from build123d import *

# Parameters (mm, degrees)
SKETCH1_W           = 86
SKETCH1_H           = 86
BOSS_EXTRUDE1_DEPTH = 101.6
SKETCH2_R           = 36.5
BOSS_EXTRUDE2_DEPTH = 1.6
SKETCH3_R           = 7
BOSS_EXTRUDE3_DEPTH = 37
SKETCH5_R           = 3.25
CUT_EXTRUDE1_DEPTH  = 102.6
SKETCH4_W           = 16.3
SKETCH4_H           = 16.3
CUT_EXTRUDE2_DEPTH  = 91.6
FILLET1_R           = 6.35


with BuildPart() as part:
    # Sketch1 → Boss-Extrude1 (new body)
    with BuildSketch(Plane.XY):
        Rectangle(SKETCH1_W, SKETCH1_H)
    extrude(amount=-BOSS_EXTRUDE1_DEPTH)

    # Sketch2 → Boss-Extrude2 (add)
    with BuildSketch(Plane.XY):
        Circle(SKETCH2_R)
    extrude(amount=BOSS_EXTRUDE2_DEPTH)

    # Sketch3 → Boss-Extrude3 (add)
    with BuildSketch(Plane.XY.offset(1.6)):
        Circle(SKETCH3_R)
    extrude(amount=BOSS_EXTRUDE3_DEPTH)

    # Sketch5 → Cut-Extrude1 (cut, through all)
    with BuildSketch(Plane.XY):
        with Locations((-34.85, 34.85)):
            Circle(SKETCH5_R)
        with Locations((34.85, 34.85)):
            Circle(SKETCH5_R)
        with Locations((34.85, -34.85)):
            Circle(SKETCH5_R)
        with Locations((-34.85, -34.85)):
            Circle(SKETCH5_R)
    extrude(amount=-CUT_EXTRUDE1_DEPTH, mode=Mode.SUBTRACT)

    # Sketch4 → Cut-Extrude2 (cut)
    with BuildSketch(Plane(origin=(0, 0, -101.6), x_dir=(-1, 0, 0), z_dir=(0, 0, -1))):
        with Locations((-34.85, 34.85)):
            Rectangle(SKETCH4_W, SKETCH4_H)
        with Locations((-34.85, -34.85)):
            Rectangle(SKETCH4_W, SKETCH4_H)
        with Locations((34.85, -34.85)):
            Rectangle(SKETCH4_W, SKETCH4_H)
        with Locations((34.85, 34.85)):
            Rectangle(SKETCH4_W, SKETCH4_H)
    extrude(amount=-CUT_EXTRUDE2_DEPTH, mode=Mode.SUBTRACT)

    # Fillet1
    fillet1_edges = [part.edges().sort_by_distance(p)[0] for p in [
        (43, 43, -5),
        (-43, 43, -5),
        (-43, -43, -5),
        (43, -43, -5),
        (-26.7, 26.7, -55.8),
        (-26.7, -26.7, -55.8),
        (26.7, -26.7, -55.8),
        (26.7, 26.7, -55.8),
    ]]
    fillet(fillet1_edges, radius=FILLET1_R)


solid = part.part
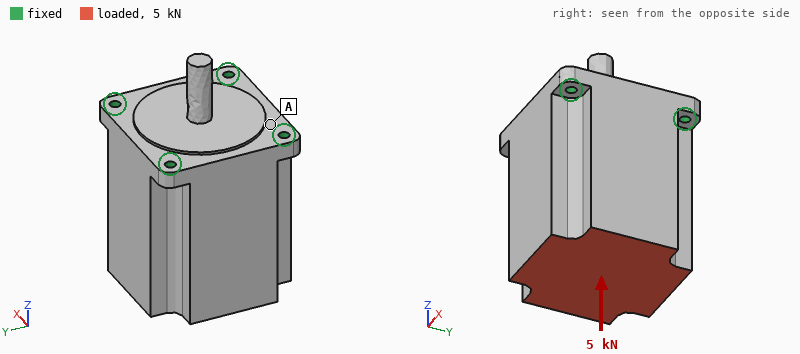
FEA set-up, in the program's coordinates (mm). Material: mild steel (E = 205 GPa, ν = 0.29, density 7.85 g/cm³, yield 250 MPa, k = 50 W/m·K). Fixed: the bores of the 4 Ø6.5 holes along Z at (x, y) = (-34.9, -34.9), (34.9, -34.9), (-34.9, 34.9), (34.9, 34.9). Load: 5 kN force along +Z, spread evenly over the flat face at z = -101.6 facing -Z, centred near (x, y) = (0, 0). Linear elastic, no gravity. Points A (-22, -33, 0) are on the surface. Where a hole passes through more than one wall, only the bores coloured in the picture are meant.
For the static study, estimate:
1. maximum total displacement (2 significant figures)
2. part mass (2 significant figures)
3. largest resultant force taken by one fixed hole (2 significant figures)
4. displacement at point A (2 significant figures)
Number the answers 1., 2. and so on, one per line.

1. 1.4 µm
2. 5.2 kg
3. 1.3 kN
4. 0.86 µm
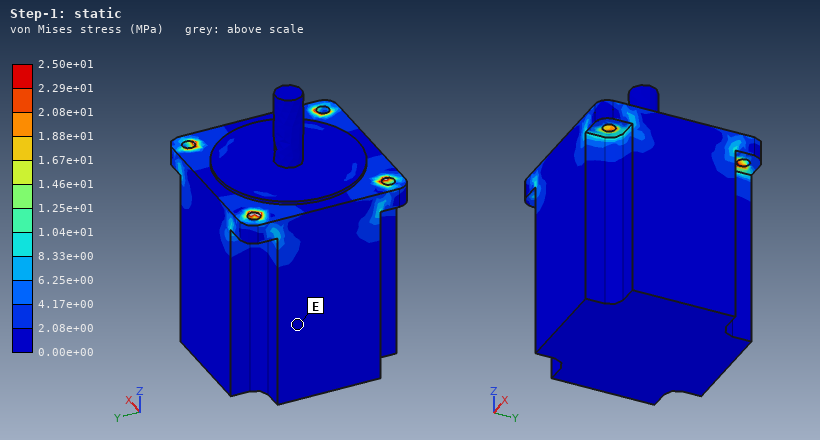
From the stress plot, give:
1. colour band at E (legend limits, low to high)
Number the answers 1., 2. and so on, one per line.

1. 0.00e+00 to 2.08e+00 MPa
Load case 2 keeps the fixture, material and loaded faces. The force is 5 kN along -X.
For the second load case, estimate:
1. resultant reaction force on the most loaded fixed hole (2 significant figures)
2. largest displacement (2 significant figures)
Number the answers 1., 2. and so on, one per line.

1. 4.0 kN
2. 13 µm
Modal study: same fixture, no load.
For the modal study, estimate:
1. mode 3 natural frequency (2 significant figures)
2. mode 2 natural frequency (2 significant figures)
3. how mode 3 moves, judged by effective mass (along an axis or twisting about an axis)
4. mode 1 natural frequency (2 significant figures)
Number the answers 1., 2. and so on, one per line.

1. 4700 Hz
2. 2500 Hz
3. along Z
4. 2500 Hz
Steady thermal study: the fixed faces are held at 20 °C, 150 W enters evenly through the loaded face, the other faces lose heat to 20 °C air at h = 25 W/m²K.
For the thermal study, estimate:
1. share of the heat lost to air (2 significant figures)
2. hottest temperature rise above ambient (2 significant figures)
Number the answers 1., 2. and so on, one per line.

1. 27 %
2. 64 K
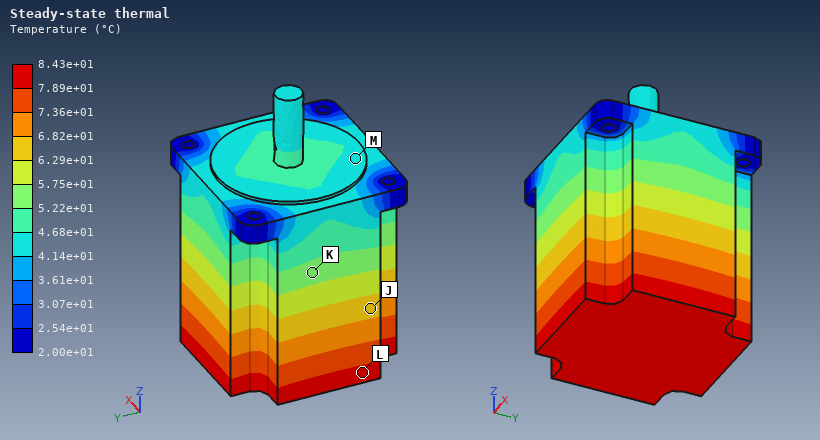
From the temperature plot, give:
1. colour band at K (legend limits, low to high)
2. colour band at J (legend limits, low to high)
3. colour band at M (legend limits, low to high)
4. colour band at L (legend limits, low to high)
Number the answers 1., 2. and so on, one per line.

1. 5.22e+01 to 5.75e+01 °C
2. 6.29e+01 to 6.82e+01 °C
3. 4.14e+01 to 4.68e+01 °C
4. 7.89e+01 to 8.43e+01 °C
